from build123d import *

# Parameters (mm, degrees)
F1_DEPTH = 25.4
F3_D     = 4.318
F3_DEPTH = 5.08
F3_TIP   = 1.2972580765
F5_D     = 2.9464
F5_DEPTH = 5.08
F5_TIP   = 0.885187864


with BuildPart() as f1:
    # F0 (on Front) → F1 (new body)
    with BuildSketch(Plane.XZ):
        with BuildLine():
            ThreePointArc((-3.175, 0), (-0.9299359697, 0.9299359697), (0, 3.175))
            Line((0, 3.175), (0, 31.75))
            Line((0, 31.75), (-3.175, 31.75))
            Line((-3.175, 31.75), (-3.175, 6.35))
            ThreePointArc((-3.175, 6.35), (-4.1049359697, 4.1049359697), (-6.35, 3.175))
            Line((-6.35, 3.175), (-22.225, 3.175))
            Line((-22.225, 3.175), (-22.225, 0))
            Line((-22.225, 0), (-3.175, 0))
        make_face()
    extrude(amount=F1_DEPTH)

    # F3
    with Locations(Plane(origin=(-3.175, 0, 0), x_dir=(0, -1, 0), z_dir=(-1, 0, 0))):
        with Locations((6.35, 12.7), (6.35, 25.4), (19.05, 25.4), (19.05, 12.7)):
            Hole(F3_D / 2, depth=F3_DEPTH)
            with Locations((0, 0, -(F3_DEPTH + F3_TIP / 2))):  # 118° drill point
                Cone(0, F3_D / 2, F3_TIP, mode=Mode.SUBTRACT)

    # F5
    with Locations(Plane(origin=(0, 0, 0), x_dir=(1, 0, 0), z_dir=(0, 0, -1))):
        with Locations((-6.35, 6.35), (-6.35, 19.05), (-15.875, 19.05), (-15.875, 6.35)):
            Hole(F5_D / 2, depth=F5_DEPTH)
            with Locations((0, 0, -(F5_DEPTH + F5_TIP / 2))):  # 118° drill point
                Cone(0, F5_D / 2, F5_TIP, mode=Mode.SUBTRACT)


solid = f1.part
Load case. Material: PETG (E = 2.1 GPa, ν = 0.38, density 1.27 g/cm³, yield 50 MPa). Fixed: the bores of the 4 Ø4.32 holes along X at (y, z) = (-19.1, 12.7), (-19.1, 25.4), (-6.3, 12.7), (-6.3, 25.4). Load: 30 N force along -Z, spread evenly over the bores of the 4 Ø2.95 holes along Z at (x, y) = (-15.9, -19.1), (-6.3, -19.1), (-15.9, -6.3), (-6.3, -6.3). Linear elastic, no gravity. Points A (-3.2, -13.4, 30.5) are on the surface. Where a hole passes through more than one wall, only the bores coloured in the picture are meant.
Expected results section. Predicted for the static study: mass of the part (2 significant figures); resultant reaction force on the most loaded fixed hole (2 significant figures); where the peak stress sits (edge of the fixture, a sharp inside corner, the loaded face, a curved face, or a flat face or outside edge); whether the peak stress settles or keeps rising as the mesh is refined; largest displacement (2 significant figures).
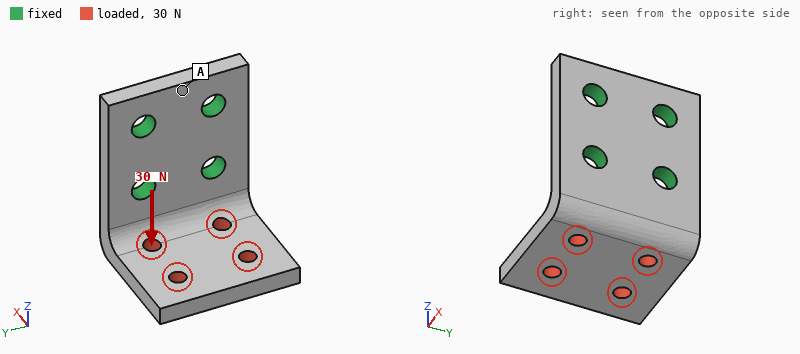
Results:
4.9 g
14 N
edge of the fixture
keeps rising
0.45 mm
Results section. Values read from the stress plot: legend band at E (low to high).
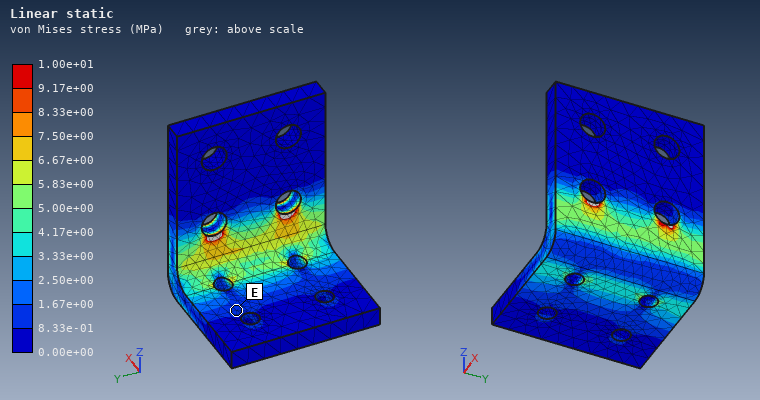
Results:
8.33e-01 to 1.67e+00 MPa
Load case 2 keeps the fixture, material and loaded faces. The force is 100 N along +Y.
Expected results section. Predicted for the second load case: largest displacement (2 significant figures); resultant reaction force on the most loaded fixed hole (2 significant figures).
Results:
0.40 mm
96 N
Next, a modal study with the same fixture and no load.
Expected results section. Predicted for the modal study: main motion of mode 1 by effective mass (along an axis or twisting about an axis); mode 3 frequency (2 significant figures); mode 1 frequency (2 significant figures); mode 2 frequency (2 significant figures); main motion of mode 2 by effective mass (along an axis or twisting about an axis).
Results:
along Z
3100 Hz
1000 Hz
1800 Hz
along Y
